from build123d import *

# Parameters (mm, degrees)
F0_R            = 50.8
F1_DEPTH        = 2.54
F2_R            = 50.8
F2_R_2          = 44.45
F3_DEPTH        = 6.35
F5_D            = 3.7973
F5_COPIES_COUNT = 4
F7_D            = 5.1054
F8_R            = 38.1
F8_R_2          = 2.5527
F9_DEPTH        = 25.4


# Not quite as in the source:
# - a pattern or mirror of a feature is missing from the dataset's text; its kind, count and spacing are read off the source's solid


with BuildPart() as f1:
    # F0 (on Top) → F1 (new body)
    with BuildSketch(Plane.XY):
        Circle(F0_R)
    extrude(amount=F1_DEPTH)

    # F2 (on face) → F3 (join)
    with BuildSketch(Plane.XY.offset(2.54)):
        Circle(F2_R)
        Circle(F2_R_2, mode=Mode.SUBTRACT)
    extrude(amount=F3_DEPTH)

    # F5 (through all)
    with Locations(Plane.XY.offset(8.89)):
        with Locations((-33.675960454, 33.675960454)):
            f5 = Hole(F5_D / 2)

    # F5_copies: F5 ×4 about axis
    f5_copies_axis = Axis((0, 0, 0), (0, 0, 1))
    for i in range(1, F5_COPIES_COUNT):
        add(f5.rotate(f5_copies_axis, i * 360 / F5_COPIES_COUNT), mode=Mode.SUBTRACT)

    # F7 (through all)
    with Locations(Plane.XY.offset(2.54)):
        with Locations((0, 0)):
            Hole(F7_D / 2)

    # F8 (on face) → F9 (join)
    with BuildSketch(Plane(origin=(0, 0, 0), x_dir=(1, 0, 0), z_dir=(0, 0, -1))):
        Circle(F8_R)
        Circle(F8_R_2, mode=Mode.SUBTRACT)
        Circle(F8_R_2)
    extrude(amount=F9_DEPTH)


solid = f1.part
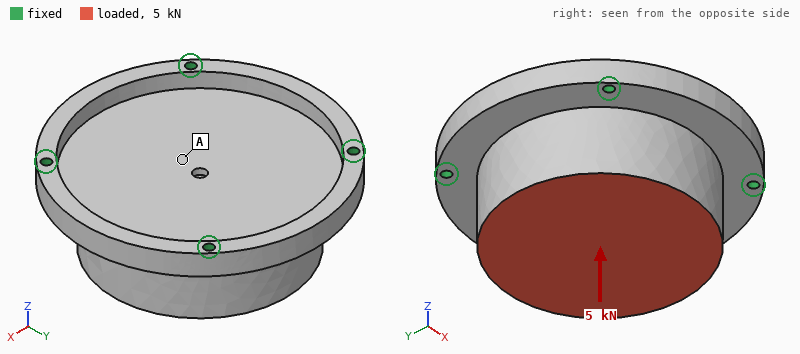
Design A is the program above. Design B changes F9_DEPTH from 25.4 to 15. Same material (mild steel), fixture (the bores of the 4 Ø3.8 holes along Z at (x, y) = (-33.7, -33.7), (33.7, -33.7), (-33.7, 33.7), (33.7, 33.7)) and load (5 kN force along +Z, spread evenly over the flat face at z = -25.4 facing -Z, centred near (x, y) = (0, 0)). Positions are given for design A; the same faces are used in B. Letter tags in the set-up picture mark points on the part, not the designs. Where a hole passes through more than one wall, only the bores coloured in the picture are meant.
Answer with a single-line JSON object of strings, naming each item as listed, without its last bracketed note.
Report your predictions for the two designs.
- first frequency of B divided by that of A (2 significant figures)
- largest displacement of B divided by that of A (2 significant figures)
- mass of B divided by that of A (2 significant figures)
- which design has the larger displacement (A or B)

{"first frequency of B divided by that of A": "1.2", "largest displacement of B divided by that of A": "1.1", "mass of B divided by that of A": "0.68", "which design has the larger displacement": "B"}
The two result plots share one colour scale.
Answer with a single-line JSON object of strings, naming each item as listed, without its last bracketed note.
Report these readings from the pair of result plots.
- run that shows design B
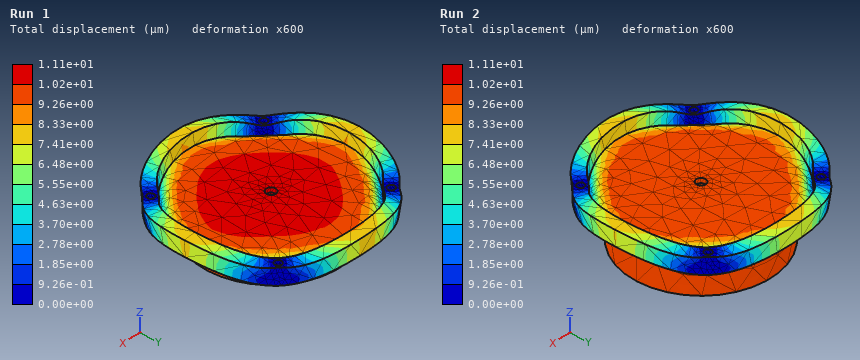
{"run that shows design B": "Run 1"}
